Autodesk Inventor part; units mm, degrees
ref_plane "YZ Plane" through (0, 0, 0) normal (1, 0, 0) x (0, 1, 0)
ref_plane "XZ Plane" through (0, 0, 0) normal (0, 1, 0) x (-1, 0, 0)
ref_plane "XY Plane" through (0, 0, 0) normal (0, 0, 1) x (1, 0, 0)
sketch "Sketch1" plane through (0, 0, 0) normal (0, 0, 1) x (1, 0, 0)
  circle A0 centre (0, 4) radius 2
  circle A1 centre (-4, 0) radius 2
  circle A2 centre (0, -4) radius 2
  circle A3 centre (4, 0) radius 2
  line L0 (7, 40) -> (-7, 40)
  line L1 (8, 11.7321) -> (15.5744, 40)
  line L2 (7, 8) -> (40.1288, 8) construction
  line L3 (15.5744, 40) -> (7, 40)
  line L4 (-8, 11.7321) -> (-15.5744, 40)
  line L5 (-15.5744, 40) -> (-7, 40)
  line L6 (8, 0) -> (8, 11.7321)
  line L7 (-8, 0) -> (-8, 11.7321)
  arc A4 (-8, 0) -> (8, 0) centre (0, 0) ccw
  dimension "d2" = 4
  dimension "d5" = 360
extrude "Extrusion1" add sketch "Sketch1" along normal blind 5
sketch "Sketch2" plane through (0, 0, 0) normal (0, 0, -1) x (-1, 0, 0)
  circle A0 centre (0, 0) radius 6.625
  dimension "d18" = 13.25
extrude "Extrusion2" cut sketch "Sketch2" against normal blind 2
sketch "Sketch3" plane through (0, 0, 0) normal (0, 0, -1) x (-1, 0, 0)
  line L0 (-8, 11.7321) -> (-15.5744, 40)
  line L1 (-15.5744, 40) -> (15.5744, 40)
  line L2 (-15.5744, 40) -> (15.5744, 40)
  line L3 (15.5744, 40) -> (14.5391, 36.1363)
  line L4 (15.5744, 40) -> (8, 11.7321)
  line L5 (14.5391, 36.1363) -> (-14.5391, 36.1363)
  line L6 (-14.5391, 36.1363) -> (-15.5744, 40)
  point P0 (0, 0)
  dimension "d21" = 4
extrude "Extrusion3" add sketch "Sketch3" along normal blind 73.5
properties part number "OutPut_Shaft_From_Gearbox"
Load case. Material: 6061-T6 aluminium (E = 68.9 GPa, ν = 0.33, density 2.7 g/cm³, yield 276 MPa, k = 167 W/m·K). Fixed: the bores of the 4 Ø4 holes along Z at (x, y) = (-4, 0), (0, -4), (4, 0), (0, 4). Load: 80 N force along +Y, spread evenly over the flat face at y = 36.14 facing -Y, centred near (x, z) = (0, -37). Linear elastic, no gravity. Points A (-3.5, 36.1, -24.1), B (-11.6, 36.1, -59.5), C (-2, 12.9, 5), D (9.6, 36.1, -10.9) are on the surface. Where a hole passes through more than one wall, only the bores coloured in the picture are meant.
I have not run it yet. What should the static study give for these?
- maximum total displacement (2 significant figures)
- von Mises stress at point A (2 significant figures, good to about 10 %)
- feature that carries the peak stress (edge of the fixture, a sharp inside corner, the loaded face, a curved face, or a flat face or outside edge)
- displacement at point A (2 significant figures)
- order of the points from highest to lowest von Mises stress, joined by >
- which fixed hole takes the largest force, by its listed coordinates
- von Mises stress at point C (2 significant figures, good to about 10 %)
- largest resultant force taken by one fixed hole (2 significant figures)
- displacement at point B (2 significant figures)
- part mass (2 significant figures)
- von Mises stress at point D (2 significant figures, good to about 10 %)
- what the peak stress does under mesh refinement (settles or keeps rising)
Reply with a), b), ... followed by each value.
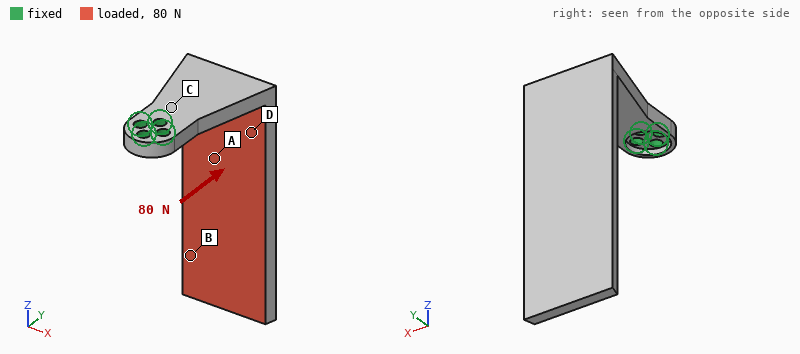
a) 1.1 mm
b) 17 MPa
c) edge of the fixture
d) 0.33 mm
e) C > D > A > B
f) (0, 4)
g) 41 MPa
h) 330 N
i) 0.83 mm
j) 35 g
k) 28 MPa
l) keeps rising
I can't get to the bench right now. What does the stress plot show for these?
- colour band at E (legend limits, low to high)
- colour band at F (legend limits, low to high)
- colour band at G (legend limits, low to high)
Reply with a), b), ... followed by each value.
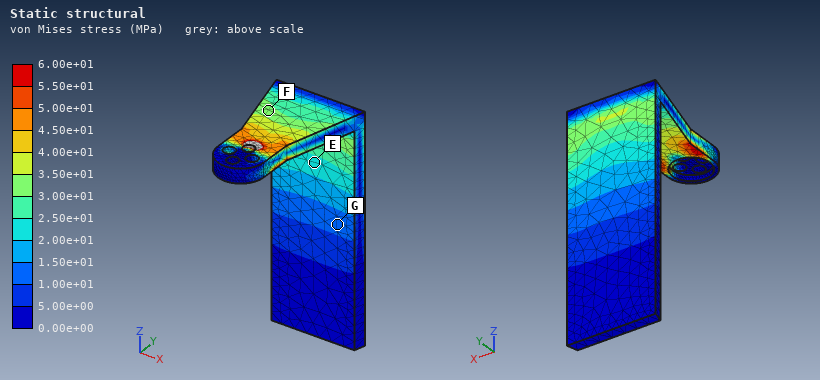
a) 2.00e+01 to 2.50e+01 MPa
b) 3.00e+01 to 3.50e+01 MPa
c) 1.00e+01 to 1.50e+01 MPa
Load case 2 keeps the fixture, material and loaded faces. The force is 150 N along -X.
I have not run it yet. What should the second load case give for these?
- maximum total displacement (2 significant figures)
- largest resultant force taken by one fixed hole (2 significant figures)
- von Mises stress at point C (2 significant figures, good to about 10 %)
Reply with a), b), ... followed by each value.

a) 0.92 mm
b) 440 N
c) 83 MPa
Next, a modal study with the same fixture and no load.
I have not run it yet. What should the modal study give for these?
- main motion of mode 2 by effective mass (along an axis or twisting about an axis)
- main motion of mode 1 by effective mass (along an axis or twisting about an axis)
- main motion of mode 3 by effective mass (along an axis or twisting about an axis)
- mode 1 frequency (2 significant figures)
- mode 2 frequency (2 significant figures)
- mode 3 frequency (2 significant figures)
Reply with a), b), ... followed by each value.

a) along X
b) along Y
c) along Z
d) 340 Hz
e) 510 Hz
f) 1200 Hz
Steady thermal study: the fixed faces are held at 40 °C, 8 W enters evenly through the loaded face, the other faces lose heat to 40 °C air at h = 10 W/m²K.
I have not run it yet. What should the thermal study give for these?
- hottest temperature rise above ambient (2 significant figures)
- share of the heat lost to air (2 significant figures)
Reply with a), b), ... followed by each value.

a) 29 K
b) 12 %
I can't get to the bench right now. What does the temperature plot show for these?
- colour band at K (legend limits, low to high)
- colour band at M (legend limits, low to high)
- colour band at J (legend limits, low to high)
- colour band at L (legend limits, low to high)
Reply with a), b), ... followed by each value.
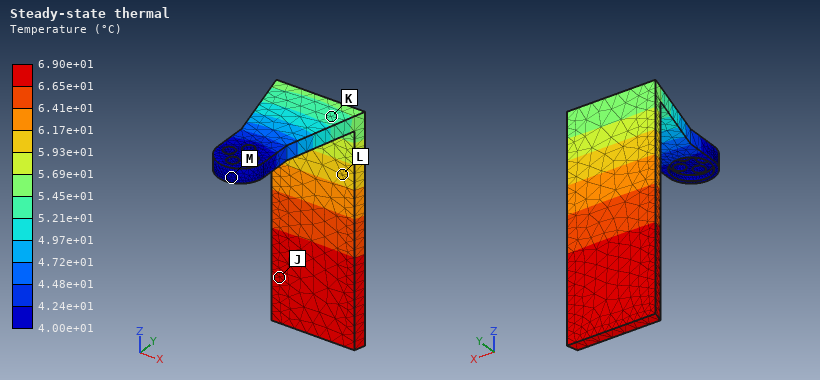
a) 5.21e+01 to 5.45e+01 °C
b) 4.00e+01 to 4.24e+01 °C
c) 6.65e+01 to 6.90e+01 °C
d) 5.93e+01 to 6.17e+01 °C
